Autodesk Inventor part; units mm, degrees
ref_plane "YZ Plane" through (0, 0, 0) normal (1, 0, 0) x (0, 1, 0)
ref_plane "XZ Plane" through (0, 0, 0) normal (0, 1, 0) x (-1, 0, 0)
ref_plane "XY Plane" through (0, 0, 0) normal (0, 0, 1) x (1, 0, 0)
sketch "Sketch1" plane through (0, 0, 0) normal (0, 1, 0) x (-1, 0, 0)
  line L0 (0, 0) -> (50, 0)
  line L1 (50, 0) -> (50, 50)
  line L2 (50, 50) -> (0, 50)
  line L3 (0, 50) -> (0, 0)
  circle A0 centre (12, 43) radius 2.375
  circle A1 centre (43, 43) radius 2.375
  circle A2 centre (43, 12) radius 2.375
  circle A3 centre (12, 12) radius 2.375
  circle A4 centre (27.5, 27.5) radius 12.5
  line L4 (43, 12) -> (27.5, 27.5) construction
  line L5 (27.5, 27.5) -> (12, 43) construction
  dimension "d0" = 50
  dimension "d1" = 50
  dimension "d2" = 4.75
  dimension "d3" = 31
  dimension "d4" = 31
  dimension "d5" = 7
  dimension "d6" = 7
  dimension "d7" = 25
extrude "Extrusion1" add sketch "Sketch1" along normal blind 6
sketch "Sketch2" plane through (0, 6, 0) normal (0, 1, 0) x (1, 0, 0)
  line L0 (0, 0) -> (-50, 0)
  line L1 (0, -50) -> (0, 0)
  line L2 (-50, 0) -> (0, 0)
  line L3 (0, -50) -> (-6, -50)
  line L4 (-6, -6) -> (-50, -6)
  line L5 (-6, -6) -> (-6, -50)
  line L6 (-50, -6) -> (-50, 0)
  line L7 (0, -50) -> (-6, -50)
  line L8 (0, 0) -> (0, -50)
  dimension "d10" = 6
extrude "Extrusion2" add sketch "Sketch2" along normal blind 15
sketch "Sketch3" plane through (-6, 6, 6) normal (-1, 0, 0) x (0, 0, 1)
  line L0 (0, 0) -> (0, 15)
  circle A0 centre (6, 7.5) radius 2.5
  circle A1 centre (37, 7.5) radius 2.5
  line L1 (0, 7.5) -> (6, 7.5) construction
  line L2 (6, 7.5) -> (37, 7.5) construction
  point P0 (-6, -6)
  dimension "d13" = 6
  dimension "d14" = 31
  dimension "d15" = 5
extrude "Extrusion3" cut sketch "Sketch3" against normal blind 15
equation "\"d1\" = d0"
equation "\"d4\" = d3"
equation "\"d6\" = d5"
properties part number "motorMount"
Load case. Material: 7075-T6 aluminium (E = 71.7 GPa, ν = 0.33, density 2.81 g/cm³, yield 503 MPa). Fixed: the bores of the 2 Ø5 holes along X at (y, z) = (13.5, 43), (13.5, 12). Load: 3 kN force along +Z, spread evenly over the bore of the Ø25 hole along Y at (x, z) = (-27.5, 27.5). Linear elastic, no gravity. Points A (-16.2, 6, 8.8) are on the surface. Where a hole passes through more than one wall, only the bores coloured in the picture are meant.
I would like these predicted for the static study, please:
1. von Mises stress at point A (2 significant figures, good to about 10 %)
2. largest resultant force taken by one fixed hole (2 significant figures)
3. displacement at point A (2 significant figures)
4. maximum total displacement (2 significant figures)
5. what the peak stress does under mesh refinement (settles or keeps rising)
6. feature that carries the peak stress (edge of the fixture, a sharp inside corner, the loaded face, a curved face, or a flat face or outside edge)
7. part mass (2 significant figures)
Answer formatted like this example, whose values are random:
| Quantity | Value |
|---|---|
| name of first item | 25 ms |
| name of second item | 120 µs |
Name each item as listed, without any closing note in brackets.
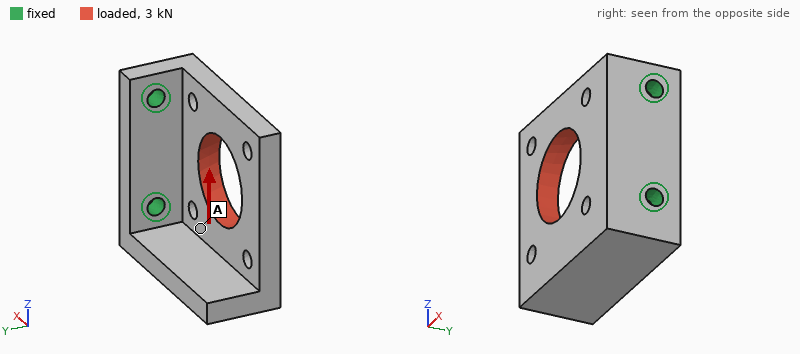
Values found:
| Quantity | Value |
|---|---|
| von Mises stress at point A | 20 MPa |
| largest resultant force taken by one fixed hole | 2.7 kN |
| displacement at point A | 0.043 mm |
| maximum total displacement | 0.16 mm |
| what the peak stress does under mesh refinement | keeps rising |
| feature that carries the peak stress | edge of the fixture |
| part mass | 56 g |
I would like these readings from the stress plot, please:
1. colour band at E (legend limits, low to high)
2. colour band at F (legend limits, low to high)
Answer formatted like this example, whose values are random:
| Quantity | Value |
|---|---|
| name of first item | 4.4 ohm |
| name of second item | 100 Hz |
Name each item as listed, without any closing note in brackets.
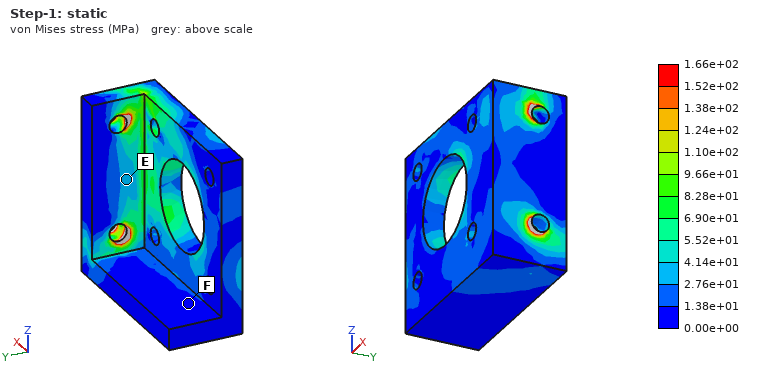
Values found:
| Quantity | Value |
|---|---|
| colour band at E | 2.76e+01 to 4.14e+01 MPa |
| colour band at F | 0.00e+00 to 1.38e+01 MPa |
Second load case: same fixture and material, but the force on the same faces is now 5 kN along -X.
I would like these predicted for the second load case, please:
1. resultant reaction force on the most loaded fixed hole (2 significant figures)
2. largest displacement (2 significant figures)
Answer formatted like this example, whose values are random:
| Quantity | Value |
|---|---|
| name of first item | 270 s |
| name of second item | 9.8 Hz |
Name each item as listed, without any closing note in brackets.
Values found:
| Quantity | Value |
|---|---|
| resultant reaction force on the most loaded fixed hole | 2.5 kN |
| largest displacement | 0.21 mm |
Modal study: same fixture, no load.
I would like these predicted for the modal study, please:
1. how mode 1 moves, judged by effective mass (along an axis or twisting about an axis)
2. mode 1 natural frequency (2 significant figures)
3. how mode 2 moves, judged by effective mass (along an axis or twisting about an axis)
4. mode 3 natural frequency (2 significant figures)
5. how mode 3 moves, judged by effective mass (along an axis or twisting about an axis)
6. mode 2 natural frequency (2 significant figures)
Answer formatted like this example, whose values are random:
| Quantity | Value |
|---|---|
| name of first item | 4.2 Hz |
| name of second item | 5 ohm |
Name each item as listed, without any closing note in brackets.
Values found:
| Quantity | Value |
|---|---|
| how mode 1 moves, judged by effective mass | along Y |
| mode 1 natural frequency | 2100 Hz |
| how mode 2 moves, judged by effective mass | along Z |
| mode 3 natural frequency | 5600 Hz |
| how mode 3 moves, judged by effective mass | along Z |
| mode 2 natural frequency | 3500 Hz |
